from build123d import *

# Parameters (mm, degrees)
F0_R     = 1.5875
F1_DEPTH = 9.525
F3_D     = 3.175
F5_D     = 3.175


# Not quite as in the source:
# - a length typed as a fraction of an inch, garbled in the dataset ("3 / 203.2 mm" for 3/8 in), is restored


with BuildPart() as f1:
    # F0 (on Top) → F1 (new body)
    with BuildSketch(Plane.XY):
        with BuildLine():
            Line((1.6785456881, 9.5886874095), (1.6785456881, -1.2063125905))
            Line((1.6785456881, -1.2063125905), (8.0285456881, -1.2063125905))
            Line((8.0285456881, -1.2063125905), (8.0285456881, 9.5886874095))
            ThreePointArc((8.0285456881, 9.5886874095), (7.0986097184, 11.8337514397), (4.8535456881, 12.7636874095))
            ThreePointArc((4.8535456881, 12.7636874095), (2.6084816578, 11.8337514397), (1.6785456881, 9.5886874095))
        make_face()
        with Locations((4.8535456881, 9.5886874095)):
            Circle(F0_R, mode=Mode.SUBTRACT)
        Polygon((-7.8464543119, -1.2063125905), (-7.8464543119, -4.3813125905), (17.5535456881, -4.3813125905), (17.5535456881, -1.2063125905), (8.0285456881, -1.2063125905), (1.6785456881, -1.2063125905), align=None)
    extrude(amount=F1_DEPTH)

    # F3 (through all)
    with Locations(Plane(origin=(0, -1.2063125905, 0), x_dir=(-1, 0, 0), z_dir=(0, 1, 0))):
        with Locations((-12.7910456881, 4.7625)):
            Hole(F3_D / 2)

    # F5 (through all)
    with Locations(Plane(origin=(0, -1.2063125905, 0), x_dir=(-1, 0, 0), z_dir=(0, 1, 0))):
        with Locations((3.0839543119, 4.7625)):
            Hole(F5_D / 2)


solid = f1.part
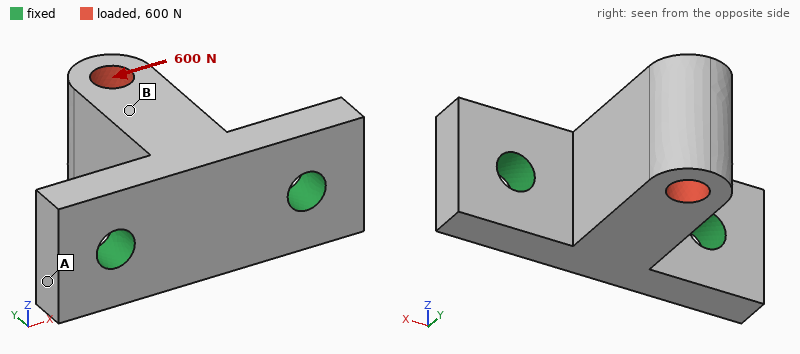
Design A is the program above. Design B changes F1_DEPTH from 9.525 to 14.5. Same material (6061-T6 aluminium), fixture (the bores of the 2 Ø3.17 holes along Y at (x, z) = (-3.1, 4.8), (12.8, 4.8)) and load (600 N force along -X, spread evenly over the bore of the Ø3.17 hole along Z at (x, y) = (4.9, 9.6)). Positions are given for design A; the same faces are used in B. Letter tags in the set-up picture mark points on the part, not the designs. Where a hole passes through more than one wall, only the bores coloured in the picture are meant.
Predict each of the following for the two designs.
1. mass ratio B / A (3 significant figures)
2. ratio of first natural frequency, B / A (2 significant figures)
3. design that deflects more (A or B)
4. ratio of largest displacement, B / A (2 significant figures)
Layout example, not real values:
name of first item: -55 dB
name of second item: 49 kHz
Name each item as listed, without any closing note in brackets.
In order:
mass ratio B / A: 1.54
ratio of first natural frequency, B / A: 0.88
design that deflects more: A
ratio of largest displacement, B / A: 0.77
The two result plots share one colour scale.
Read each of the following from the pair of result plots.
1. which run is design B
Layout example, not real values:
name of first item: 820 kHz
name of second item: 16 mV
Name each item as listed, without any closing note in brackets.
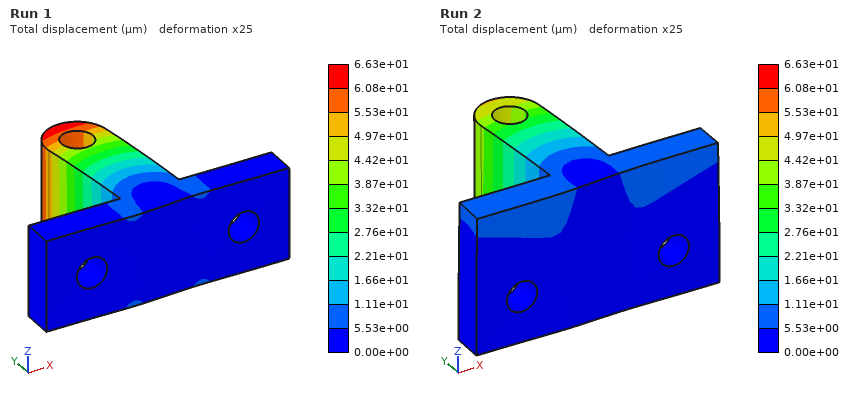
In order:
which run is design B: Run 2
